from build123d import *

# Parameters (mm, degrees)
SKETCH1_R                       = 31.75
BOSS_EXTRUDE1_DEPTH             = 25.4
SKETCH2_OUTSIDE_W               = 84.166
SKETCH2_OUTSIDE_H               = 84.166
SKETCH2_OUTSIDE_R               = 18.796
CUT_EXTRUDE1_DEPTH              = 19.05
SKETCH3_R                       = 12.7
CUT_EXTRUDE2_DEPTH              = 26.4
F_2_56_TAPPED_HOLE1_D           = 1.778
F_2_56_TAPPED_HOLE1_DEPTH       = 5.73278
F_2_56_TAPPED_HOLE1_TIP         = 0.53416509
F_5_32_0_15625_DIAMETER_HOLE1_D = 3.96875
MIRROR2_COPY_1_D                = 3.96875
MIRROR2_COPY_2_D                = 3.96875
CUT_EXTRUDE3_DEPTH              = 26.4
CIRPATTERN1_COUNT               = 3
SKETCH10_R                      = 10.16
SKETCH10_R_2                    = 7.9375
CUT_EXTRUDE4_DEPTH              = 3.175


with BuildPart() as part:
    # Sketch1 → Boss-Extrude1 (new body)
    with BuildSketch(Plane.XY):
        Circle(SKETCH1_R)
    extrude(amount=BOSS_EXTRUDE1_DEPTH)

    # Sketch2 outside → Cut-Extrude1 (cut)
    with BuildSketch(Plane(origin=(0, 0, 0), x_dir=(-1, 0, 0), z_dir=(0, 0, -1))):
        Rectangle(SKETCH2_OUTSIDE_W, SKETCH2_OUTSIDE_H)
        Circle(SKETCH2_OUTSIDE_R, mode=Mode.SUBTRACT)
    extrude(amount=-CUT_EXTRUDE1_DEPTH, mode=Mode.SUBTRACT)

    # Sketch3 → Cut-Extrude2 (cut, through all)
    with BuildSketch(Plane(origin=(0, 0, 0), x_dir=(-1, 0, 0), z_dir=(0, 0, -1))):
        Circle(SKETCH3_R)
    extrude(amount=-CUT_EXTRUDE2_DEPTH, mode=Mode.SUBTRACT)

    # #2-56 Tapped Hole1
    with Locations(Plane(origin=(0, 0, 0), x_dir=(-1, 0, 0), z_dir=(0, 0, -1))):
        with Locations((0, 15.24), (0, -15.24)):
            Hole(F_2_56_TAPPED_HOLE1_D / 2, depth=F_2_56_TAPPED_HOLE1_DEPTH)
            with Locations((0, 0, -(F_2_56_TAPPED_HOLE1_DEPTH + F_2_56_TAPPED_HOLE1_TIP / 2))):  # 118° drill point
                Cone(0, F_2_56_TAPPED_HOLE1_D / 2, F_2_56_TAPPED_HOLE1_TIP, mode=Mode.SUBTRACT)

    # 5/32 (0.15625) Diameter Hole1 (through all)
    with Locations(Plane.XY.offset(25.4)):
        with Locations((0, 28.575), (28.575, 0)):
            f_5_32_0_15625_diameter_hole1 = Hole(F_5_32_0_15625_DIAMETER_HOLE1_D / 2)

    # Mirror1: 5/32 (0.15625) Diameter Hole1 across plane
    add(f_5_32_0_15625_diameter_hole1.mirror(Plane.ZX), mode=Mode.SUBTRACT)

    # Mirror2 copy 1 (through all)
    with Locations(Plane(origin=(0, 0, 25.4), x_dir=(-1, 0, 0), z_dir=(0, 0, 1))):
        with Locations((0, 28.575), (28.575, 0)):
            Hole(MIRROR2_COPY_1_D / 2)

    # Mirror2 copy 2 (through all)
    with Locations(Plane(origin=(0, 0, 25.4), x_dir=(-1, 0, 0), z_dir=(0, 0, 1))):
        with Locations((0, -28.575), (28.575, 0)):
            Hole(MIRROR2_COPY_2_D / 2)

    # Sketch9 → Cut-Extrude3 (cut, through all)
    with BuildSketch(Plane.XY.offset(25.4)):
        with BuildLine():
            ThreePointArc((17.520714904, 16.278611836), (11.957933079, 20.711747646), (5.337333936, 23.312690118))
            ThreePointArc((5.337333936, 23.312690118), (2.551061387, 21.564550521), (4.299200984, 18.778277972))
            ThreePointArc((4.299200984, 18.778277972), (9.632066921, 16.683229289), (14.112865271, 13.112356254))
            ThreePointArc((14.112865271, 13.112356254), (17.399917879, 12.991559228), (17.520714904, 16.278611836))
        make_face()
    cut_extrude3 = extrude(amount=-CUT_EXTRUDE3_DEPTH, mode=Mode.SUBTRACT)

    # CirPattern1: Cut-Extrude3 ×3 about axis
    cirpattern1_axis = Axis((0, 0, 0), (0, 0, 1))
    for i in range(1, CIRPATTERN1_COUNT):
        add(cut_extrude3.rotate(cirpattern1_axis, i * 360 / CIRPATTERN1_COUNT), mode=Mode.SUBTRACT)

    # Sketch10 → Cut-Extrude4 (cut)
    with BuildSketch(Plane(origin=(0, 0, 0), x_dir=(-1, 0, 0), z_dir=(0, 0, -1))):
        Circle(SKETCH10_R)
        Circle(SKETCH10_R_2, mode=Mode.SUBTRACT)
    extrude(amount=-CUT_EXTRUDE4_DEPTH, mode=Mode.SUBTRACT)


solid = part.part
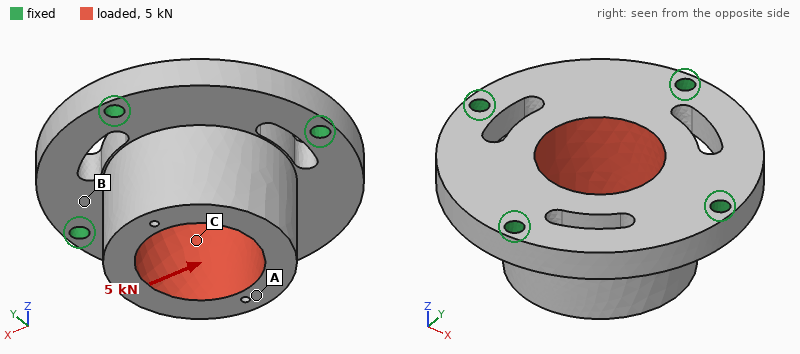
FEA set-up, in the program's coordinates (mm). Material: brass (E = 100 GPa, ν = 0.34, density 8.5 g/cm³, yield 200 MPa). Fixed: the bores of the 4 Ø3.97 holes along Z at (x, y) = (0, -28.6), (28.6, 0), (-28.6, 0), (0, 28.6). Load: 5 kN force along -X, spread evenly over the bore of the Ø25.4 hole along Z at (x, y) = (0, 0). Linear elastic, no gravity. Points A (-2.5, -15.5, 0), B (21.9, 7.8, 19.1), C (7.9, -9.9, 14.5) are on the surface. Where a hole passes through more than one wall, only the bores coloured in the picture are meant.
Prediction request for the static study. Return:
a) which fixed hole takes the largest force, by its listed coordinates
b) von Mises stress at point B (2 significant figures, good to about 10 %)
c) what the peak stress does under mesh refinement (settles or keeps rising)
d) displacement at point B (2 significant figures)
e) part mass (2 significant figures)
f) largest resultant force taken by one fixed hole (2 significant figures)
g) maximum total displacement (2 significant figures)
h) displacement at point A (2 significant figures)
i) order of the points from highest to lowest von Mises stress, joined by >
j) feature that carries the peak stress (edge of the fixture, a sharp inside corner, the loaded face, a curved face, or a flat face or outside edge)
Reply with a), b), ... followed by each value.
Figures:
a) (28.6, 0)
b) 25 MPa
c) keeps rising
d) 4.2 µm
e) 230 g
f) 2.2 kN
g) 25 µm
h) 18 µm
i) B > C > A
j) edge of the fixture
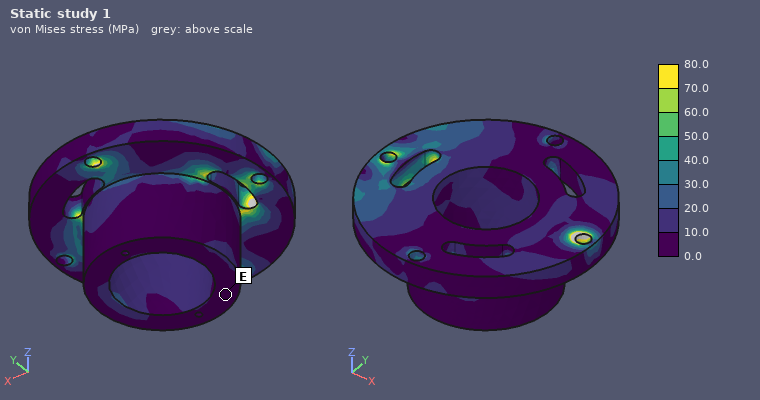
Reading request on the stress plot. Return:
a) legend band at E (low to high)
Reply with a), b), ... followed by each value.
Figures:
a) 0.0 to 10.0 MPa
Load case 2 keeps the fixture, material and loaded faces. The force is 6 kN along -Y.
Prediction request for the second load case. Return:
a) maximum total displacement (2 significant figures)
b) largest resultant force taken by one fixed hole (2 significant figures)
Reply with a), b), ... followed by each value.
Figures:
a) 22 µm
b) 2.1 kN
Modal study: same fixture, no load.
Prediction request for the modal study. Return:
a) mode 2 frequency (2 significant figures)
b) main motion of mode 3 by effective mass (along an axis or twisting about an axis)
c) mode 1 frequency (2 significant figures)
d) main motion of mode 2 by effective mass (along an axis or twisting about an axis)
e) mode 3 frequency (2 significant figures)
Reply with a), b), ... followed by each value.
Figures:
a) 7600 Hz
b) along Z
c) 6200 Hz
d) along Y
e) 8100 Hz
